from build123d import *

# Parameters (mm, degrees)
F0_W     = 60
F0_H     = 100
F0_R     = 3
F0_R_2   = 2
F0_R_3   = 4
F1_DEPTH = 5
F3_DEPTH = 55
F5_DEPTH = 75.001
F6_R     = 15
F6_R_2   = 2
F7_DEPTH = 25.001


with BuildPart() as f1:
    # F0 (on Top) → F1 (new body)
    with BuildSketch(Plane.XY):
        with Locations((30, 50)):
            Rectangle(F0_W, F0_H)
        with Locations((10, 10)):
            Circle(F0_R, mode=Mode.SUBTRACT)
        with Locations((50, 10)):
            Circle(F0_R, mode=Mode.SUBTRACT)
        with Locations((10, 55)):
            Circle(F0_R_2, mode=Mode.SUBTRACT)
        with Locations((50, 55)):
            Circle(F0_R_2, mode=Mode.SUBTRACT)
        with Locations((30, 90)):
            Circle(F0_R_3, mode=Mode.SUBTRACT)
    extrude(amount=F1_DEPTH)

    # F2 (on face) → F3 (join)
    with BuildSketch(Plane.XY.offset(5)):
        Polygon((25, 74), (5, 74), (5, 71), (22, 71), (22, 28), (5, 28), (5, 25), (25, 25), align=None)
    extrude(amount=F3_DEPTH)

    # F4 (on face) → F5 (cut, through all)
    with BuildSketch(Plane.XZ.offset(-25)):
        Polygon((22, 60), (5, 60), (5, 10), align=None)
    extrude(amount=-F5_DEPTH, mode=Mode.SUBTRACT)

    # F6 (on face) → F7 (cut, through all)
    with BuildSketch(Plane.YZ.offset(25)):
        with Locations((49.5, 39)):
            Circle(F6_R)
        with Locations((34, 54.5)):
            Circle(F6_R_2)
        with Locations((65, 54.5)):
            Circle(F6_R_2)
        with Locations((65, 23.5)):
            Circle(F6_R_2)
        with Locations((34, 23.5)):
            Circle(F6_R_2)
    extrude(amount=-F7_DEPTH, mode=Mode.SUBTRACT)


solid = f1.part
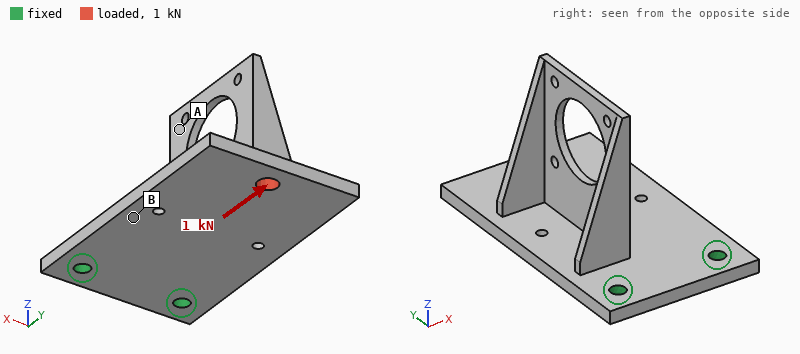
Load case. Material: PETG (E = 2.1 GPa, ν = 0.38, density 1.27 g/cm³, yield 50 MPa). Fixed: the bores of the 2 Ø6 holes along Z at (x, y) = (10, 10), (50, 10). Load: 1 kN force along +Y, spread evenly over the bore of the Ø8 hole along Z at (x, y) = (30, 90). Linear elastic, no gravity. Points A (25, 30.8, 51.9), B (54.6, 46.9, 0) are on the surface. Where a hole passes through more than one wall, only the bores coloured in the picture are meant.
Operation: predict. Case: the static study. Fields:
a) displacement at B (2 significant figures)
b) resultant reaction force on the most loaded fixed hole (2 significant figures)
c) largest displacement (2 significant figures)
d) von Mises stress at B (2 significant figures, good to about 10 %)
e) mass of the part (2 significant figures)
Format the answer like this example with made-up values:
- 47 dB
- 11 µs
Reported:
- 0.079 mm
- 510 N
- 0.31 mm
- 3.5 MPa
- 49 g
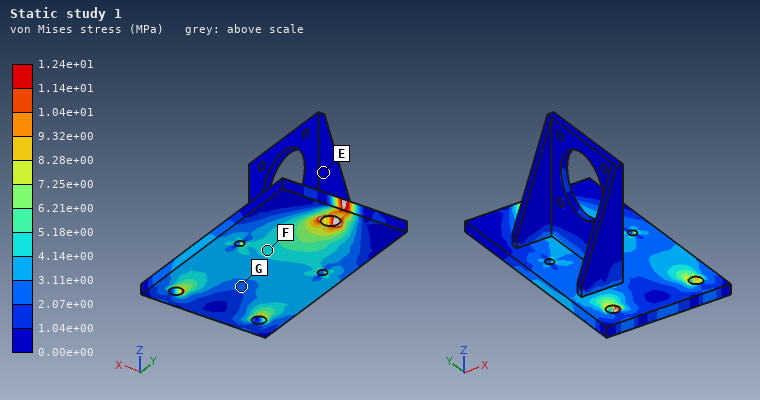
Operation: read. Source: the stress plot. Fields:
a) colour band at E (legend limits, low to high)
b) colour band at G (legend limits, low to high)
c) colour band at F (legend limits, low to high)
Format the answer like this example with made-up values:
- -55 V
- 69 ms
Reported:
- 0.00e+00 to 1.04e+00 MPa
- 2.07e+00 to 3.11e+00 MPa
- 4.14e+00 to 5.18e+00 MPa
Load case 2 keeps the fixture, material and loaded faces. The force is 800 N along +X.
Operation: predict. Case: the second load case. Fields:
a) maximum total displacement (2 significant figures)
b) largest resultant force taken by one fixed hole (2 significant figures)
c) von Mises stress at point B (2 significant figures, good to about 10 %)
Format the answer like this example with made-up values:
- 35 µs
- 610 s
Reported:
- 1.4 mm
- 1.5 kN
- 8.9 MPa
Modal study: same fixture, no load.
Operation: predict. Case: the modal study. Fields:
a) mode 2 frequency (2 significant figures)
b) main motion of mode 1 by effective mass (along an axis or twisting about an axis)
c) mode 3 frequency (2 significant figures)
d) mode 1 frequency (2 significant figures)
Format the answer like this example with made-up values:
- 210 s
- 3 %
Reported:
- 340 Hz
- along Z
- 770 Hz
- 130 Hz
